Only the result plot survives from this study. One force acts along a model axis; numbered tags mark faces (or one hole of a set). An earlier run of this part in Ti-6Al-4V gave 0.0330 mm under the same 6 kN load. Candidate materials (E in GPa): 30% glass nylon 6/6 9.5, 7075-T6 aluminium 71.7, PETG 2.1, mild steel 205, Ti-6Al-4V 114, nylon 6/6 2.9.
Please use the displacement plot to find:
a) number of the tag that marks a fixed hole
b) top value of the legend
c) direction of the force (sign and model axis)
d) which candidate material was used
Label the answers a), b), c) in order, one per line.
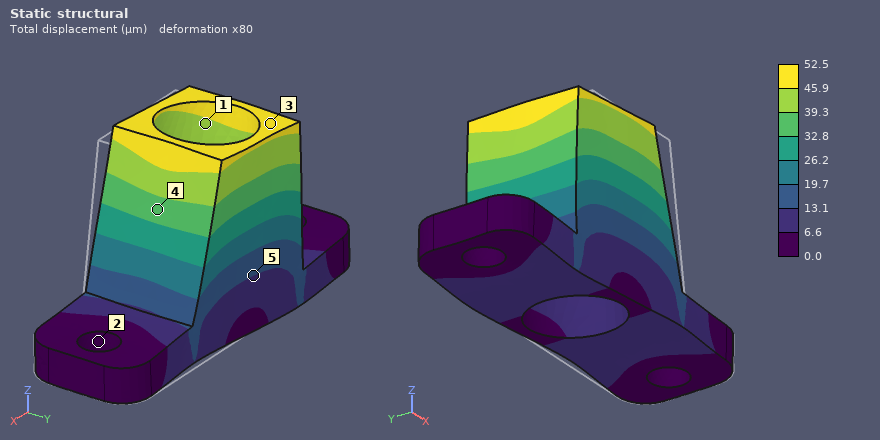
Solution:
a) 2
b) 52.5 µm
c) -X
d) 7075-T6 aluminium
